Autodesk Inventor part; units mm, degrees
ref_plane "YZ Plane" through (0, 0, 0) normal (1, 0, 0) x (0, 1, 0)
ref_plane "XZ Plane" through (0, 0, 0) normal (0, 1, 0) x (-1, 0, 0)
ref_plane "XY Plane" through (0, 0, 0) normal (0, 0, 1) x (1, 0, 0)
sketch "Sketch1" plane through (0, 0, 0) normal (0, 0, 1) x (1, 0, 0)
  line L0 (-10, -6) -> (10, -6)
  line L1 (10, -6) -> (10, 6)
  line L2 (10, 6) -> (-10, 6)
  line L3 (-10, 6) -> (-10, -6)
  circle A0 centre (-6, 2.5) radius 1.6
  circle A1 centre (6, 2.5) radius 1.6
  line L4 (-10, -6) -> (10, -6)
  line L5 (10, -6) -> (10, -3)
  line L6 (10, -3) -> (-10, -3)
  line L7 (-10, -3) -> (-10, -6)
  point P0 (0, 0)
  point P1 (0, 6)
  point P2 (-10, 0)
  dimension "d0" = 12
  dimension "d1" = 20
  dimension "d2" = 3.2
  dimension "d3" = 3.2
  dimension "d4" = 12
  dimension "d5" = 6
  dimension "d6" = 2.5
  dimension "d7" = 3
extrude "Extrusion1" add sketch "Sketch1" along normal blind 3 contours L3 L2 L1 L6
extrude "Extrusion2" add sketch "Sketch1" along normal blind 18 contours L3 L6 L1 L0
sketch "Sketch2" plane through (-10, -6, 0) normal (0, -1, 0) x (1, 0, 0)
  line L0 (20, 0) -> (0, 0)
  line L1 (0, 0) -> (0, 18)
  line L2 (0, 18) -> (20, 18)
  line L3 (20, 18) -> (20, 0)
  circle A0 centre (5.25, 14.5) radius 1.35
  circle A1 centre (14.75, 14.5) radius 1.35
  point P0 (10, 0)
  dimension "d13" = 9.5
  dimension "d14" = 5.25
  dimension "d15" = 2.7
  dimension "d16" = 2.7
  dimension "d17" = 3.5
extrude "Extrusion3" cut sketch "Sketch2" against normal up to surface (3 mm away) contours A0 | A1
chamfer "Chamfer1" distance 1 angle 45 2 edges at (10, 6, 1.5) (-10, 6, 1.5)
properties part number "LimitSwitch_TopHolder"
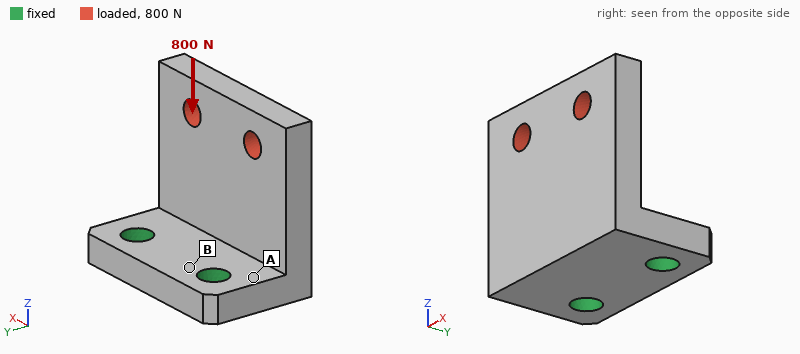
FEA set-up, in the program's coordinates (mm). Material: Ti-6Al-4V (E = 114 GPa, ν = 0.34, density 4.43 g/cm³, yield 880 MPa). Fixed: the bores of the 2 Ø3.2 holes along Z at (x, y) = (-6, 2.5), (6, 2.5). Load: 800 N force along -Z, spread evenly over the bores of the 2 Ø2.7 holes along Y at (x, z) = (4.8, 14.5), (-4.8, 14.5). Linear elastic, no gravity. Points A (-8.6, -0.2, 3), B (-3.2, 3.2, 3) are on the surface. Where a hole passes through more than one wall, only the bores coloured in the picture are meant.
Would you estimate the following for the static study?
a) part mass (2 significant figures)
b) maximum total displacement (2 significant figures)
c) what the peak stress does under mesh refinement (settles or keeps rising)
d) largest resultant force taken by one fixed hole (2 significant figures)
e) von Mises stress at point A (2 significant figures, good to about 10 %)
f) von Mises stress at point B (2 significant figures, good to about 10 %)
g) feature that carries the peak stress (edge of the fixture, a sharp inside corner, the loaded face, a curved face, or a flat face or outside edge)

6.8 g
58 µm
keeps rising
400 N
98 MPa
46 MPa
edge of the fixture
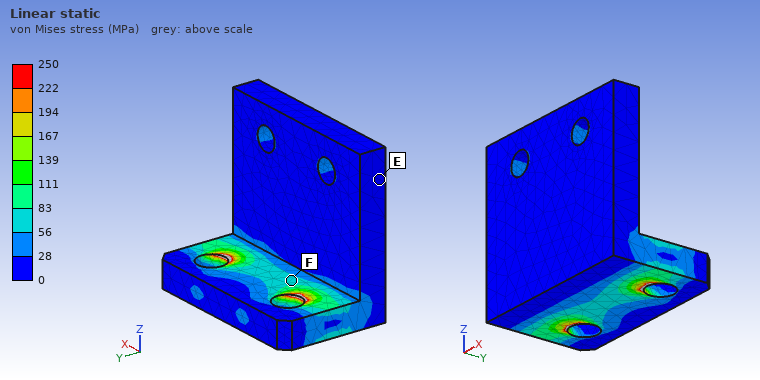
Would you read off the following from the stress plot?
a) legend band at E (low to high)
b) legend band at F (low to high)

0 to 28 MPa
56 to 83 MPa
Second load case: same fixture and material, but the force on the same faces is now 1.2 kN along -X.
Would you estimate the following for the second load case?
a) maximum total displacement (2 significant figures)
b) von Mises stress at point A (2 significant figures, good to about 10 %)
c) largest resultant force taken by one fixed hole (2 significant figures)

92 µm
190 MPa
1.4 kN
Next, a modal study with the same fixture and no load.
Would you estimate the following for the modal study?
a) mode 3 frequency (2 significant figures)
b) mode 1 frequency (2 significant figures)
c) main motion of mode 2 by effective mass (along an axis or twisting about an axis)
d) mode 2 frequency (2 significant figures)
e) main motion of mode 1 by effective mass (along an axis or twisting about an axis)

18 kHz
6000 Hz
along X
12 kHz
along Y
